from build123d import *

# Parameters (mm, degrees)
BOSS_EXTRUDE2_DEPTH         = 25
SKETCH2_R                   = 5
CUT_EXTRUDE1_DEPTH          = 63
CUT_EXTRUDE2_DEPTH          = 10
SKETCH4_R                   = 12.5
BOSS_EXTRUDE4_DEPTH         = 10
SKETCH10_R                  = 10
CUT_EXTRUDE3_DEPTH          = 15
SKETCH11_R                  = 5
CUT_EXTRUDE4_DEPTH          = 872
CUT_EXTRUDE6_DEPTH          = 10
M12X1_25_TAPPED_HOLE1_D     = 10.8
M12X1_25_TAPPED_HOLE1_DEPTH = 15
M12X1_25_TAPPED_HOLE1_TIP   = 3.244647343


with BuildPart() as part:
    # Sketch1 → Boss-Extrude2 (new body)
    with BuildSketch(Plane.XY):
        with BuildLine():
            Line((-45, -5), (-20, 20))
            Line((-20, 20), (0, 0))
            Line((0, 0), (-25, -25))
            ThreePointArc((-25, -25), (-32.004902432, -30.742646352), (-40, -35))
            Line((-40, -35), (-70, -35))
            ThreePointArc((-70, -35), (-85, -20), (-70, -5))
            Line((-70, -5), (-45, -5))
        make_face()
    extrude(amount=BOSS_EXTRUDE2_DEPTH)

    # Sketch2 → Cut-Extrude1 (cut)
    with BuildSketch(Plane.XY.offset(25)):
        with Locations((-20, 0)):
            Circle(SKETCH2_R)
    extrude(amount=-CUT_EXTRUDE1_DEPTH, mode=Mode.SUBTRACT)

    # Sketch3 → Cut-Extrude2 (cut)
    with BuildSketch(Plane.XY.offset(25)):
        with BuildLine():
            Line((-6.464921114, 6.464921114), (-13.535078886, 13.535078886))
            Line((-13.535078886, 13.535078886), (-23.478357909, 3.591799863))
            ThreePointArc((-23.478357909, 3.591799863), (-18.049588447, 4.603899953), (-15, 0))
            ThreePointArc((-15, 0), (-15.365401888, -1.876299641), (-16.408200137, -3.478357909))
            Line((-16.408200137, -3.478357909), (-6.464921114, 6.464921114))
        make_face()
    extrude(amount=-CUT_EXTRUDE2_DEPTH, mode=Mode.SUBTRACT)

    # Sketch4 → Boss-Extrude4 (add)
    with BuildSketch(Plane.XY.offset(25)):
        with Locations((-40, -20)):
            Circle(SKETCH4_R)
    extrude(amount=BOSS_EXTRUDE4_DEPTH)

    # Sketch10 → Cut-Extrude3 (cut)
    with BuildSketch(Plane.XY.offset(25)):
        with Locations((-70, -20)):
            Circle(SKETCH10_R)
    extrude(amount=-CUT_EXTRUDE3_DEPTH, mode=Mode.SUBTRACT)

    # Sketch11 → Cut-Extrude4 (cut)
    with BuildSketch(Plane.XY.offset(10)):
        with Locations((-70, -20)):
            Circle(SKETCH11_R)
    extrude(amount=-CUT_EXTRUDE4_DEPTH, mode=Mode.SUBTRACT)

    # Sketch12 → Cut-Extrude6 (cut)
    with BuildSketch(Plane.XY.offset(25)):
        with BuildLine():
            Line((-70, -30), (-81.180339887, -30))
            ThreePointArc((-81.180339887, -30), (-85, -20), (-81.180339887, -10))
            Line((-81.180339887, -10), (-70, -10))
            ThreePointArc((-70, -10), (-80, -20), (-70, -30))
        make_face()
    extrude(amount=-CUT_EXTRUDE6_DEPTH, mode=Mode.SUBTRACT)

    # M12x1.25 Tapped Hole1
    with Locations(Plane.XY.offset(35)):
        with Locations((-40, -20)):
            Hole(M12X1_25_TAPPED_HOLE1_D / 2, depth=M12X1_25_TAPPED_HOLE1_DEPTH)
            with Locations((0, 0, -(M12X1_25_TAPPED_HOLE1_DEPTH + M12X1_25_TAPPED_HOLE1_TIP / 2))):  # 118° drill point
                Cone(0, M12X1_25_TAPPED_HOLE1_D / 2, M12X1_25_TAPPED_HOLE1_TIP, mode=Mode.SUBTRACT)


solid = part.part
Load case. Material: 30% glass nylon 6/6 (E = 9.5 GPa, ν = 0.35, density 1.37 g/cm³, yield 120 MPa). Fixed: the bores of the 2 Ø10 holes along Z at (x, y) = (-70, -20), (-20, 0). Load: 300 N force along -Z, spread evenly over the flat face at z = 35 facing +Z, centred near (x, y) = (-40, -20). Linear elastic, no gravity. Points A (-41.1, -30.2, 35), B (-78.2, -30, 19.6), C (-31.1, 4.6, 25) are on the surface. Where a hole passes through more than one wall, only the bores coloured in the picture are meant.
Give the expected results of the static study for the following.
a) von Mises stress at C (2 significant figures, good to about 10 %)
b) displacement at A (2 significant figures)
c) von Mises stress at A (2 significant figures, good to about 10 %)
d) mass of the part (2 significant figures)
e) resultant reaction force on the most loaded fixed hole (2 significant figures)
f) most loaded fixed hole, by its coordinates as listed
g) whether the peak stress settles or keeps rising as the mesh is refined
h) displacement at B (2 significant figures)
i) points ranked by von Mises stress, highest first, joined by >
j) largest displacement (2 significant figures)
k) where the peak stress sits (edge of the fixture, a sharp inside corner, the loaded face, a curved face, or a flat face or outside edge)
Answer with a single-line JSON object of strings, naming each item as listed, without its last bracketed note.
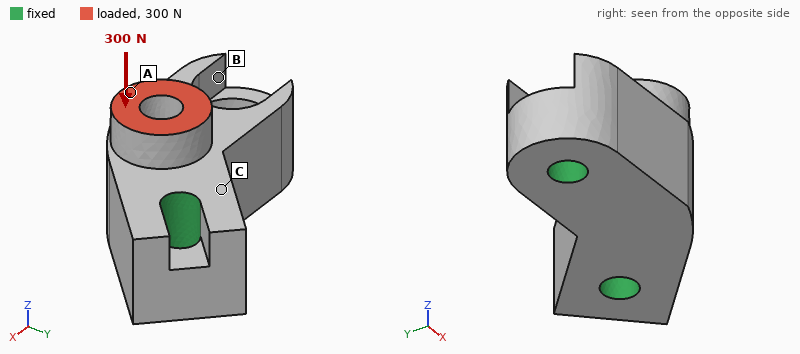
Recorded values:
{"von Mises stress at C": "0.44 MPa", "displacement at A": "7.6 µm", "von Mises stress at A": "0.75 MPa", "mass of the part": "75 g", "resultant reaction force on the most loaded fixed hole": "190 N", "most loaded fixed hole, by its coordinates as listed": "(-20, 0)", "whether the peak stress settles or keeps rising as the mesh is refined": "keeps rising", "displacement at B": "1.9 µm", "points ranked by von Mises stress, highest first, joined by >": "A > C > B", "largest displacement": "8.1 µm", "where the peak stress sits": "edge of the fixture"}
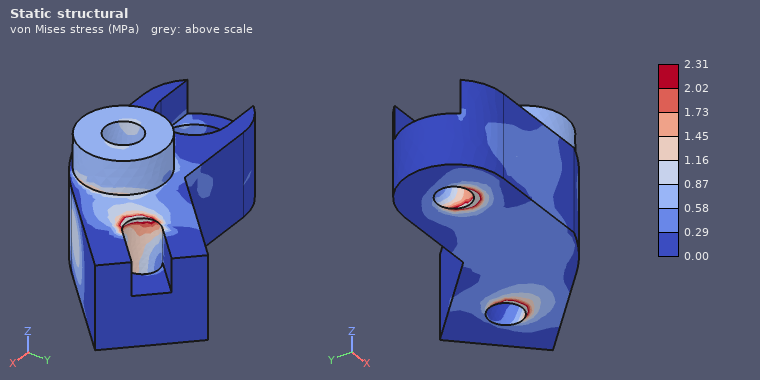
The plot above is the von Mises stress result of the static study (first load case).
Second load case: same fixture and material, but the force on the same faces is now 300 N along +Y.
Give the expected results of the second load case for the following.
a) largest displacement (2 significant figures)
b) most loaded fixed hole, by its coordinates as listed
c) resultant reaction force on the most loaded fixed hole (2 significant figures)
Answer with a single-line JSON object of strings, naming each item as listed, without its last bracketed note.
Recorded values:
{"largest displacement": "23 µm", "most loaded fixed hole, by its coordinates as listed": "(-20, 0)", "resultant reaction force on the most loaded fixed hole": "250 N"}
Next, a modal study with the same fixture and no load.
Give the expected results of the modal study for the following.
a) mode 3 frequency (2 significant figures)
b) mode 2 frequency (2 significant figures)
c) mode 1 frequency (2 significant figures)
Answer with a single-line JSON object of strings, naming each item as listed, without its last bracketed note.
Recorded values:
{"mode 3 frequency": "12 kHz", "mode 2 frequency": "9400 Hz", "mode 1 frequency": "5900 Hz"}
